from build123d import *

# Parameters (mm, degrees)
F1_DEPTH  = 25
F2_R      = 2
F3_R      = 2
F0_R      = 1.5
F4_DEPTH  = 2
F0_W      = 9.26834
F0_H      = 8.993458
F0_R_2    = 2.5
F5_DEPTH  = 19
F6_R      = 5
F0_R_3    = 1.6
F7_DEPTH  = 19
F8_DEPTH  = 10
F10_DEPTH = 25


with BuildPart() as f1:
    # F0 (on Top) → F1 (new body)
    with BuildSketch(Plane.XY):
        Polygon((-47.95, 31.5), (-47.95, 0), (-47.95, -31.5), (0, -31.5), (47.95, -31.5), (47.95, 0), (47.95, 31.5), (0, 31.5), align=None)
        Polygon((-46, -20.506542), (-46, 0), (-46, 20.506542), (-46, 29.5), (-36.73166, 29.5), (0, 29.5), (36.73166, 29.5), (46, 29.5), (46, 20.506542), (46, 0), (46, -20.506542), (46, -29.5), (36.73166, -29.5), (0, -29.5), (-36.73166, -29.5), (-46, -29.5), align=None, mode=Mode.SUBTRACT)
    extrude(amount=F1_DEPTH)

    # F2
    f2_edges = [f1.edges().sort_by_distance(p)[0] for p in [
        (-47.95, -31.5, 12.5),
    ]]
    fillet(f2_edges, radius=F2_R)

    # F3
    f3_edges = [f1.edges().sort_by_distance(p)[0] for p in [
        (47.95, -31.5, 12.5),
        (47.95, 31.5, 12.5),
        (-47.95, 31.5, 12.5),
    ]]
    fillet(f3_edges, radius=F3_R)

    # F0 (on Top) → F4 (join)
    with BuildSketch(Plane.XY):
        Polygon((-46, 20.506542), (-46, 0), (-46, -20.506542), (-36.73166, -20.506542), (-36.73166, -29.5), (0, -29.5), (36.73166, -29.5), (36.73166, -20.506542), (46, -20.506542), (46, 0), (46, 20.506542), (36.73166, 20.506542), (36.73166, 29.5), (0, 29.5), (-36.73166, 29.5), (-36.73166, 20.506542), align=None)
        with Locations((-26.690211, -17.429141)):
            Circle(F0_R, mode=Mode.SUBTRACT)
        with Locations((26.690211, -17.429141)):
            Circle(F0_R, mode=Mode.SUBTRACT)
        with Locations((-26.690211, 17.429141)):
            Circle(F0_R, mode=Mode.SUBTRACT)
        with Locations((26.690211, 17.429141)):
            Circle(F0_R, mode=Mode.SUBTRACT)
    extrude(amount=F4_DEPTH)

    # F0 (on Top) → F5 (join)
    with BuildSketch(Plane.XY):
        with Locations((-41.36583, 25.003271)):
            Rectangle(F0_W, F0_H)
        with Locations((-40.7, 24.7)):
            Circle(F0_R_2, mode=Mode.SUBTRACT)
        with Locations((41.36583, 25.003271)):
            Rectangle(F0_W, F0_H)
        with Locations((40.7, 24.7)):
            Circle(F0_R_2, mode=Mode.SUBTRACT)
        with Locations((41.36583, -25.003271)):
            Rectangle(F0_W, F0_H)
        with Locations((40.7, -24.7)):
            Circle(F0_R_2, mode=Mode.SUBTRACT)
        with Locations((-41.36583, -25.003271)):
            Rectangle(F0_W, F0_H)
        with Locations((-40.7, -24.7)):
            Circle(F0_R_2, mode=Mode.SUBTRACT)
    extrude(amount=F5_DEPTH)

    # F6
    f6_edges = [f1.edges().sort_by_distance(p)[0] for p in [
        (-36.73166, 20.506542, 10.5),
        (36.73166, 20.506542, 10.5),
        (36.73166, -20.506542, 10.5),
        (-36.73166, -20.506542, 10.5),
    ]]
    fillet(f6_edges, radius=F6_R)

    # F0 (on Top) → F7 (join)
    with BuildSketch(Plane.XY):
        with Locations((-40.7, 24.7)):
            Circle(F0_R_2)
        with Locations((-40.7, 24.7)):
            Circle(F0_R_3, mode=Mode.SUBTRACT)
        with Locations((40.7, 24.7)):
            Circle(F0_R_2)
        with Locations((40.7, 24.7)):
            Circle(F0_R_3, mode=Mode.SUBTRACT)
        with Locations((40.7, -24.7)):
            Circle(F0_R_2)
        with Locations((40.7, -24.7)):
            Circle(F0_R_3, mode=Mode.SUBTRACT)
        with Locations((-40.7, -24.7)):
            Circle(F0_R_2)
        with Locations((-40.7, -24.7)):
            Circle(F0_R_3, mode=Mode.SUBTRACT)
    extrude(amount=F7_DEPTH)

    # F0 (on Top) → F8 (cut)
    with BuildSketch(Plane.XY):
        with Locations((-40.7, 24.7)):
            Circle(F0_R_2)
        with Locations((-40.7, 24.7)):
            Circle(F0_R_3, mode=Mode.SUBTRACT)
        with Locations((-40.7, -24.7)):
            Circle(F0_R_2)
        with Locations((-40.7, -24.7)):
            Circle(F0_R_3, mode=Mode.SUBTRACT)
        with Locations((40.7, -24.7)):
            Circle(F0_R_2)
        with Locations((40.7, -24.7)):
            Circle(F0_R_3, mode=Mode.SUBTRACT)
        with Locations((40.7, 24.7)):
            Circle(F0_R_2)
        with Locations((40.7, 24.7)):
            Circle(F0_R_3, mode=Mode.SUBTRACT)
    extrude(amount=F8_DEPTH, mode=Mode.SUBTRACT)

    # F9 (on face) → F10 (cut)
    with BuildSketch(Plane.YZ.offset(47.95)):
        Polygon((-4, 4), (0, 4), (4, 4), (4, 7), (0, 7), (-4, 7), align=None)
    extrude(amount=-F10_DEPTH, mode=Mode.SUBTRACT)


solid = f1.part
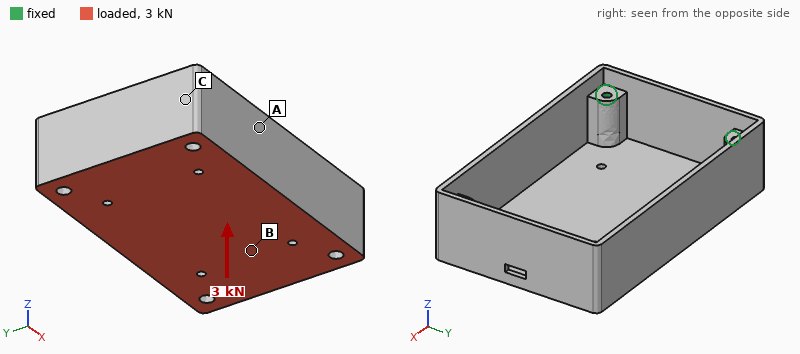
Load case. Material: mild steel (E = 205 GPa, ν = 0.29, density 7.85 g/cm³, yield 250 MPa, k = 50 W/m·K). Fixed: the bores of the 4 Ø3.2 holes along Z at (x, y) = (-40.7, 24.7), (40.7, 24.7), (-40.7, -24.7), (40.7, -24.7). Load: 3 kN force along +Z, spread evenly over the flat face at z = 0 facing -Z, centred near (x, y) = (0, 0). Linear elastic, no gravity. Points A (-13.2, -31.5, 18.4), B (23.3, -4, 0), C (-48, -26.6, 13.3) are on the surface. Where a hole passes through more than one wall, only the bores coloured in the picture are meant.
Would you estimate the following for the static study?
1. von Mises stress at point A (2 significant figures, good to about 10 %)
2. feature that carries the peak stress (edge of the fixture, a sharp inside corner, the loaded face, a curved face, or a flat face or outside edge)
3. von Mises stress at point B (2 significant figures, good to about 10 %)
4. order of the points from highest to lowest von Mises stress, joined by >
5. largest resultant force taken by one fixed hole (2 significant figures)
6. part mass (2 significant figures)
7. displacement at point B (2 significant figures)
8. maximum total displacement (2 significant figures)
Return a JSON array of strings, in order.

["43 MPa", "a curved face", "84 MPa", "B > A > C", "860 N", "240 g", "0.12 mm", "0.18 mm"]
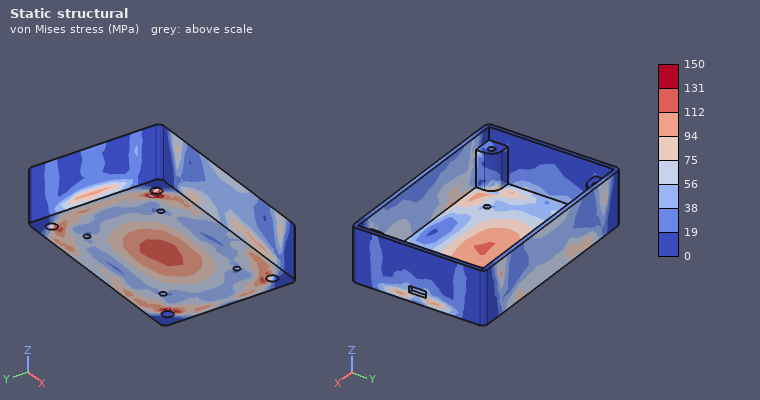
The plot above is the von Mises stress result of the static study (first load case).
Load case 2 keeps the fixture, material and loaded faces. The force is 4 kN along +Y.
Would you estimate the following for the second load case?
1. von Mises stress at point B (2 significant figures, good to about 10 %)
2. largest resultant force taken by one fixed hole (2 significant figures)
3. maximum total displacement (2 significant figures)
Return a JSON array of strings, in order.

["15 MPa", "1.1 kN", "10 µm"]
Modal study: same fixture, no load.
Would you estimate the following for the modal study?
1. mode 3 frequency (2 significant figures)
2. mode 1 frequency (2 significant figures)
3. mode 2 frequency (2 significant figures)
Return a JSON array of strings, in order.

["4000 Hz", "2400 Hz", "3300 Hz"]
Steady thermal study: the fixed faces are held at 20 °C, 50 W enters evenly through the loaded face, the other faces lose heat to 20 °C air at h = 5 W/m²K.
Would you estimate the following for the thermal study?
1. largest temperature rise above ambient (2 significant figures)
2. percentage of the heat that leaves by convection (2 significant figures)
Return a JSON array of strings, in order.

["73 K", "6.6 %"]
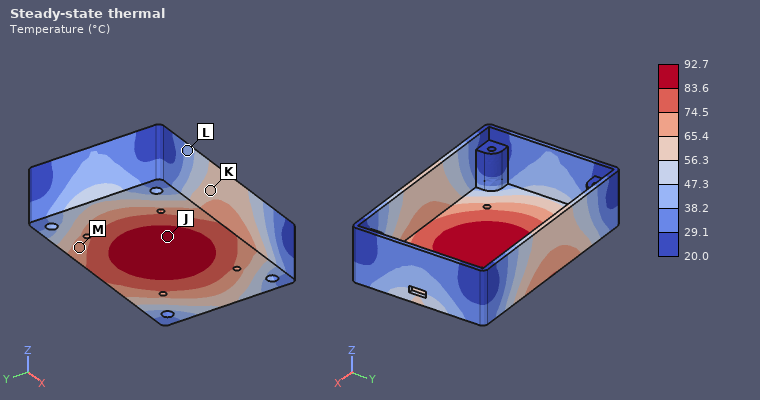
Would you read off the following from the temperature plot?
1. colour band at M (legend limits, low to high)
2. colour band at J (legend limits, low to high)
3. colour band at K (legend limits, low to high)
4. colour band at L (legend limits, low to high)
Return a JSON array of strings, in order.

["65.4 to 74.5 °C", "83.6 to 92.7 °C", "56.3 to 65.4 °C", "38.2 to 47.3 °C"]
